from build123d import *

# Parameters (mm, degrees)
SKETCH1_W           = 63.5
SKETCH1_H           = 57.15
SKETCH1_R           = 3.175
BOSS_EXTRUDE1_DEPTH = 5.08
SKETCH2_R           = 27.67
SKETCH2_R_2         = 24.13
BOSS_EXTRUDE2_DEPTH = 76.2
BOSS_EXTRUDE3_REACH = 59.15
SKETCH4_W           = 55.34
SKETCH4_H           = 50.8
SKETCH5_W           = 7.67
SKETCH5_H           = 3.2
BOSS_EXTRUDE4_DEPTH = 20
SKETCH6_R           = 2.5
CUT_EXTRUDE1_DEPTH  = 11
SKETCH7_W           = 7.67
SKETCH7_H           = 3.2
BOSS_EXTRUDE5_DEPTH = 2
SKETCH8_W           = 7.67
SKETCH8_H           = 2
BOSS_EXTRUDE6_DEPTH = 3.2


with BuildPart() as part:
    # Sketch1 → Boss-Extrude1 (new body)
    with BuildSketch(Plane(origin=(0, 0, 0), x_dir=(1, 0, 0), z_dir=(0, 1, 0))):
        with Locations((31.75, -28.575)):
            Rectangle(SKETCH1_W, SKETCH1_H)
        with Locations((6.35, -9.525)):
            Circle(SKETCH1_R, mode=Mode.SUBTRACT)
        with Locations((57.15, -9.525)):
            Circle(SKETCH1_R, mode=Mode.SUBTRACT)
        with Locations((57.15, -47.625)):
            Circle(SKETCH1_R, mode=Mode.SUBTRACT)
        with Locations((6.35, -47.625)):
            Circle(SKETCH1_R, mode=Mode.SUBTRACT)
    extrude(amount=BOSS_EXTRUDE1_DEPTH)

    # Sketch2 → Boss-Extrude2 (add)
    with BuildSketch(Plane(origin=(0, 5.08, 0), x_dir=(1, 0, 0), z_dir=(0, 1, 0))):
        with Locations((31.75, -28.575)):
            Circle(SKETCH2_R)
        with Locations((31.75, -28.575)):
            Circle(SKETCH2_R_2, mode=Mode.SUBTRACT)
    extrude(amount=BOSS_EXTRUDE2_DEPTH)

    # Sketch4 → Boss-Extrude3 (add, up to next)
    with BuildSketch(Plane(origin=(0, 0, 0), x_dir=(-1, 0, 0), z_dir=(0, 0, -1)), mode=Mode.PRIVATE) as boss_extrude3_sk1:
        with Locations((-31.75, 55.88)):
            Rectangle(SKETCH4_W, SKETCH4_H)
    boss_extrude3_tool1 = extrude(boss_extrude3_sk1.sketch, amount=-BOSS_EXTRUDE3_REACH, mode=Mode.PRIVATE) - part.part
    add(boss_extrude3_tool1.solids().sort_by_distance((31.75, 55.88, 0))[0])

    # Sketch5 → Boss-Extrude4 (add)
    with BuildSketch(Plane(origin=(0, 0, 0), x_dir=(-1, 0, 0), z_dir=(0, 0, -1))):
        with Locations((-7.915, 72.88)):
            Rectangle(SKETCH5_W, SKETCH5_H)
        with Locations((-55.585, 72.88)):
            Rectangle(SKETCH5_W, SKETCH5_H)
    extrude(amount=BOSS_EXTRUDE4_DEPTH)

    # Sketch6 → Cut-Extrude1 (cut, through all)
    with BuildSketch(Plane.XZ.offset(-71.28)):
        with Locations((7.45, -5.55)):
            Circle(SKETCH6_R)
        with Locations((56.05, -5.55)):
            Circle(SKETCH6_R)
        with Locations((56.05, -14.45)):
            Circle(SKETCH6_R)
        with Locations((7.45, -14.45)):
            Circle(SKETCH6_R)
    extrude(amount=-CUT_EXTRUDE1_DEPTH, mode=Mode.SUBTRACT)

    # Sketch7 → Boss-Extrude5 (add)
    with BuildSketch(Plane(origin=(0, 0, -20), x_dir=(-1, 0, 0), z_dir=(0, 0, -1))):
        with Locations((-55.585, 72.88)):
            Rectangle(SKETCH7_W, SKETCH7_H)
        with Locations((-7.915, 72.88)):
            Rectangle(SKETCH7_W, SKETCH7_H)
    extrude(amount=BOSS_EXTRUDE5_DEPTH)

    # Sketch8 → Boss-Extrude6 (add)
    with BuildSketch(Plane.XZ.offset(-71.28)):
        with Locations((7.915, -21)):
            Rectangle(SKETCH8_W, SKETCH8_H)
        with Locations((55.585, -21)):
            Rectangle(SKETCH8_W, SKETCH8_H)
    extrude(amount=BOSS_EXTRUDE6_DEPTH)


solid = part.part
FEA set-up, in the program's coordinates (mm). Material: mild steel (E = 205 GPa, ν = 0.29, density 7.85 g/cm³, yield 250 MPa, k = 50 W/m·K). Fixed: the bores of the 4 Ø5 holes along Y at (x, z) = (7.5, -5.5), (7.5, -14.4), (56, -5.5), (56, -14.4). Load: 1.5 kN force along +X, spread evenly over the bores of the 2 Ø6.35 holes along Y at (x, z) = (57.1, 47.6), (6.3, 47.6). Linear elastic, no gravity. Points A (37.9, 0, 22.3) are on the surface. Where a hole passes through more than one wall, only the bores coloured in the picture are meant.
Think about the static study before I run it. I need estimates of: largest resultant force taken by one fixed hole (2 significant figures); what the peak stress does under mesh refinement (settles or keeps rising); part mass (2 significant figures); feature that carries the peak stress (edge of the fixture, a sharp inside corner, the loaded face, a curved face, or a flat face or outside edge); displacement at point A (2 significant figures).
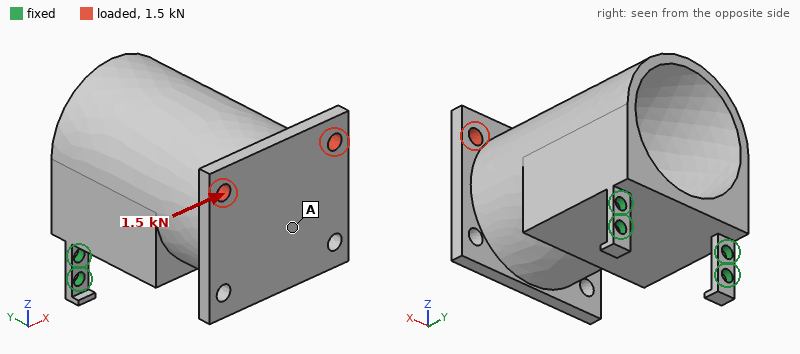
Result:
2.8 kN
keeps rising
640 g
edge of the fixture
51 µm
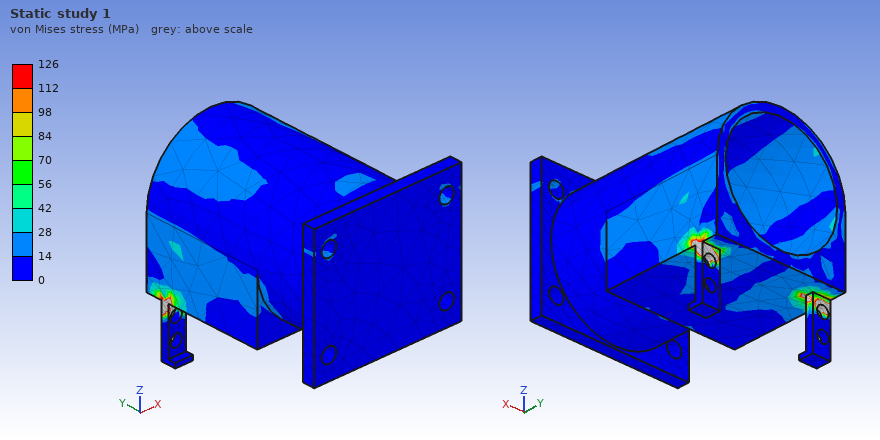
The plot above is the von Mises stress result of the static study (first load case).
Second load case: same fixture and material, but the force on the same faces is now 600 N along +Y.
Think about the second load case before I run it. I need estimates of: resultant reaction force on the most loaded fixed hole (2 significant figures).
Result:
320 N
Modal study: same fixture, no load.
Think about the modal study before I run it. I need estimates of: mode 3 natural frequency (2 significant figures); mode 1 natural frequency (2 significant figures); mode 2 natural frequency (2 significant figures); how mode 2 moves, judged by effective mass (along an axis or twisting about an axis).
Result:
2300 Hz
160 Hz
1600 Hz
along X
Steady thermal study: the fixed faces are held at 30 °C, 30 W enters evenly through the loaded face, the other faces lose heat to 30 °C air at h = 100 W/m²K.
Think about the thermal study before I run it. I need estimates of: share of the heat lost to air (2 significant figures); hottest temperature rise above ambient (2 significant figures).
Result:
97 %
50 K
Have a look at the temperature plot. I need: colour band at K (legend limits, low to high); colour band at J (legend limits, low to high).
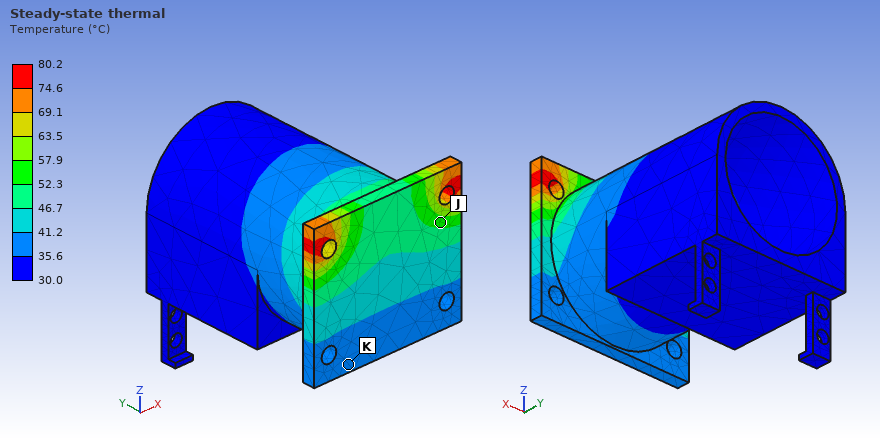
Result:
35.6 to 41.2 °C
52.3 to 57.9 °C
